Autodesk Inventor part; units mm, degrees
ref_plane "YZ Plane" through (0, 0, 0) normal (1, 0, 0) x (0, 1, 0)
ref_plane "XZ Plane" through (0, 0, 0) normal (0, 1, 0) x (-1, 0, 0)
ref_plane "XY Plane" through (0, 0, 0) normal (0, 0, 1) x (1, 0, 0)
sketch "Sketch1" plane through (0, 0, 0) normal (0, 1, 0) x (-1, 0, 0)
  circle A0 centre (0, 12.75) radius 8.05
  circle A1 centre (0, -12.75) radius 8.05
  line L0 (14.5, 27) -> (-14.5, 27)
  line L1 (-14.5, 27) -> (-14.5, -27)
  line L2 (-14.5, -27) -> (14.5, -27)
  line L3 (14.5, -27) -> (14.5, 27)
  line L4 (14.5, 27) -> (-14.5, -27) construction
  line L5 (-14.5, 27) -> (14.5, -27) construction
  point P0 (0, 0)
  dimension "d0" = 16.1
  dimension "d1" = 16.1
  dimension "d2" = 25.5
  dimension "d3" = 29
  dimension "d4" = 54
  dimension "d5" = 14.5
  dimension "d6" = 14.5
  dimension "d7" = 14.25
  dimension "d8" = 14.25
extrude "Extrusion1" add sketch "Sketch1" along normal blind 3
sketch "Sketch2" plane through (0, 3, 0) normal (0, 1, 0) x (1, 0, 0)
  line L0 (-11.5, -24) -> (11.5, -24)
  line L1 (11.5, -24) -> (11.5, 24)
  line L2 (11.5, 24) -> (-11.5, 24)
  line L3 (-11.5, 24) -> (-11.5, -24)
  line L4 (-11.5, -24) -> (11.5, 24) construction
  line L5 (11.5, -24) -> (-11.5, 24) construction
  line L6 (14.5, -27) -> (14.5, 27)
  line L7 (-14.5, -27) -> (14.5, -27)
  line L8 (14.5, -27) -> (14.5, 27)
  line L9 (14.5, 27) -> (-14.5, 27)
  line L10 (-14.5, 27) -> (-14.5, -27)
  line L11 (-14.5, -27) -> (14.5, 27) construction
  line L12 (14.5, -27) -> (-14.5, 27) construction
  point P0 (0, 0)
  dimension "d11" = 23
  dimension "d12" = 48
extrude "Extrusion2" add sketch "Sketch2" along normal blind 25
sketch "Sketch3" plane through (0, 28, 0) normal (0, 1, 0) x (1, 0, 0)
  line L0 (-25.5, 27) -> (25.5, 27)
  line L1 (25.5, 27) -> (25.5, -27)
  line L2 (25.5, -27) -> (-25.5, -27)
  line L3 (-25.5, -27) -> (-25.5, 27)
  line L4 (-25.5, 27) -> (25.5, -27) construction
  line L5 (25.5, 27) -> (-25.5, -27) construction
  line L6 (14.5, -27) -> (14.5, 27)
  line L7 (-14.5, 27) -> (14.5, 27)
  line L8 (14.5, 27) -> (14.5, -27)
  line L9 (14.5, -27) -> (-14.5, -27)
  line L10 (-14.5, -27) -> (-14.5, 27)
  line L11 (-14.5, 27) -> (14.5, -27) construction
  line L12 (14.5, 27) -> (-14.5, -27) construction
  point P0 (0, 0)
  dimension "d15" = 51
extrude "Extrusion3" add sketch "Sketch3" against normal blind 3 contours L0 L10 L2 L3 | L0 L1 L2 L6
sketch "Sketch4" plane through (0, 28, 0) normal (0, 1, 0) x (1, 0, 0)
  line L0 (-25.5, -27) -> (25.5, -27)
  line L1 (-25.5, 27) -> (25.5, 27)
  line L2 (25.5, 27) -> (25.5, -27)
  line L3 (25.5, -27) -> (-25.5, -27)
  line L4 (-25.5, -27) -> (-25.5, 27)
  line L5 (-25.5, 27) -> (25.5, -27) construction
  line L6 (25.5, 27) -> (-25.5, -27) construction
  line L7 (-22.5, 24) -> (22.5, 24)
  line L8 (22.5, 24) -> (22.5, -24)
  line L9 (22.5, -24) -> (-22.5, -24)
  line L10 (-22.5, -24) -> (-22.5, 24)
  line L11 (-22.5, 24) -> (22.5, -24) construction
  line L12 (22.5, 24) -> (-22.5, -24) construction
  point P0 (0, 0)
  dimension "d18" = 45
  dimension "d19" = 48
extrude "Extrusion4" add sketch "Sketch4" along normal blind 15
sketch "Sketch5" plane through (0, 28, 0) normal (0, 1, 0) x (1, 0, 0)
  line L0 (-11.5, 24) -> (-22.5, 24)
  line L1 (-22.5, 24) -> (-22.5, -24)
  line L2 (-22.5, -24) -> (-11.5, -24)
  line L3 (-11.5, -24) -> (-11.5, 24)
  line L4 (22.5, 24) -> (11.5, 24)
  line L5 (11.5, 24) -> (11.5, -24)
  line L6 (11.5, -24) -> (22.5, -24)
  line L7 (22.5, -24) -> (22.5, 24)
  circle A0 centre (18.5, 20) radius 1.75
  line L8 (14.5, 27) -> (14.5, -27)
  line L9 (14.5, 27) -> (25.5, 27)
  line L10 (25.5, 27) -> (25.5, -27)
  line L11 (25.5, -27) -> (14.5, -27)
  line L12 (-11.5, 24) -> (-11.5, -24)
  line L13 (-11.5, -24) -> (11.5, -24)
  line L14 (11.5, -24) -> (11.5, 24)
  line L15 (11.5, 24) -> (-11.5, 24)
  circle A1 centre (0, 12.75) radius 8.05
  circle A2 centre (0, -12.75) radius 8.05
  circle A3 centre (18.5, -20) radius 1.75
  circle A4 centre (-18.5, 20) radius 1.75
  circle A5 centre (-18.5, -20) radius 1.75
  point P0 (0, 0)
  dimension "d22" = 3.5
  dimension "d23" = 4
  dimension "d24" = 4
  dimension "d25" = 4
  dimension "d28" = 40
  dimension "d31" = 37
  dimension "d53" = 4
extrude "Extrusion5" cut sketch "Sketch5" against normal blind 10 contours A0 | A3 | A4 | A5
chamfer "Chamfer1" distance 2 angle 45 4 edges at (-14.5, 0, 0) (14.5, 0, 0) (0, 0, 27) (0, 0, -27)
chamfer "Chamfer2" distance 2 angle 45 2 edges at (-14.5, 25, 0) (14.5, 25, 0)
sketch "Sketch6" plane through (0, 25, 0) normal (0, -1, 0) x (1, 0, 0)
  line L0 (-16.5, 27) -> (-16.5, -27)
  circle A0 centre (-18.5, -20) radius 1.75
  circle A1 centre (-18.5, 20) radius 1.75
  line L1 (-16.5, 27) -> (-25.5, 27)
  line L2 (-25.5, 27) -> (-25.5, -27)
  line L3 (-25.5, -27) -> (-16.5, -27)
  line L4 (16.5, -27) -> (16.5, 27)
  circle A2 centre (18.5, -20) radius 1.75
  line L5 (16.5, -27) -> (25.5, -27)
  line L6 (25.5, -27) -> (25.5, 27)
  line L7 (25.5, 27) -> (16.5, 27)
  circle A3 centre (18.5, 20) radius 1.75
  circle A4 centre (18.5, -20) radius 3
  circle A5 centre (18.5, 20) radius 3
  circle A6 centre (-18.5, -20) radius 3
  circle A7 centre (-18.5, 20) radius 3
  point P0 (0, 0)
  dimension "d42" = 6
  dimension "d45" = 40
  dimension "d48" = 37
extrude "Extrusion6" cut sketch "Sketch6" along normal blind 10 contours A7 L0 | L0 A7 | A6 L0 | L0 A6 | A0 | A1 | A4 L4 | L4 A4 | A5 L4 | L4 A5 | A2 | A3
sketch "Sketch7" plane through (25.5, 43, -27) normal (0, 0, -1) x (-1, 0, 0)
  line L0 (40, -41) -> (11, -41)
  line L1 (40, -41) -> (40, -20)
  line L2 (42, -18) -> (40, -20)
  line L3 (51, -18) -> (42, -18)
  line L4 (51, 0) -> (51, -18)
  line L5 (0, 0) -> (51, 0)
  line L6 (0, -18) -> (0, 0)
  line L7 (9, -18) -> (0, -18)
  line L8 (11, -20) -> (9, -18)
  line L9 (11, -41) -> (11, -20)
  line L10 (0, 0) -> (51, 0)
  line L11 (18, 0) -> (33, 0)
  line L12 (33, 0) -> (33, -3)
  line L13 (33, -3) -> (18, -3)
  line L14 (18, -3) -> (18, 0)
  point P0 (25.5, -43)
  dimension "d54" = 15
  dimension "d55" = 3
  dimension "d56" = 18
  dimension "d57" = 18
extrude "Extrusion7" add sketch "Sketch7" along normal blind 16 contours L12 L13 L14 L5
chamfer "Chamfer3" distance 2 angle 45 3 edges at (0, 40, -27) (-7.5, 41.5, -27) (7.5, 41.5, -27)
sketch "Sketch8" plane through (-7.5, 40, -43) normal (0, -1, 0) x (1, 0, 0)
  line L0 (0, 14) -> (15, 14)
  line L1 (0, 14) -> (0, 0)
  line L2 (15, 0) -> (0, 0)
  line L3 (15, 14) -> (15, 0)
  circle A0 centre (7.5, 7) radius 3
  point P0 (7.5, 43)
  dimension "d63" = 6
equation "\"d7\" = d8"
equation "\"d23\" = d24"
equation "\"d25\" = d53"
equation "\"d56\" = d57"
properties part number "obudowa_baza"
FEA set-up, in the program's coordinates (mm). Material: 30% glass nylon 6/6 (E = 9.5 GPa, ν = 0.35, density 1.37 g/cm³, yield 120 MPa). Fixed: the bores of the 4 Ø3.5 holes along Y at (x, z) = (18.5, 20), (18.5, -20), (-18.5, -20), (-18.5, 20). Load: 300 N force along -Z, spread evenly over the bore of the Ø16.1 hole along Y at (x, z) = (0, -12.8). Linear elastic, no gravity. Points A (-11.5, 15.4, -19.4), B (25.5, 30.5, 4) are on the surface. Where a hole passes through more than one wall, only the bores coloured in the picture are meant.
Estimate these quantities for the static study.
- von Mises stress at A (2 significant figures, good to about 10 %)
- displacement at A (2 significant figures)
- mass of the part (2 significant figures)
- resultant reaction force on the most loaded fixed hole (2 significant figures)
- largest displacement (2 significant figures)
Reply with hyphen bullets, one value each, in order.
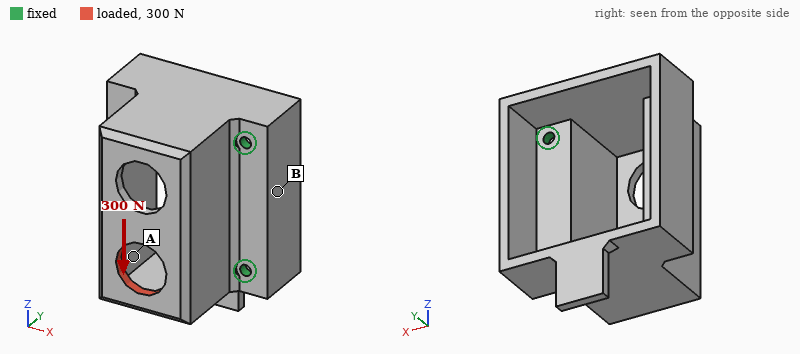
- 1.9 MPa
- 9.3 µm
- 38 g
- 120 N
- 28 µm
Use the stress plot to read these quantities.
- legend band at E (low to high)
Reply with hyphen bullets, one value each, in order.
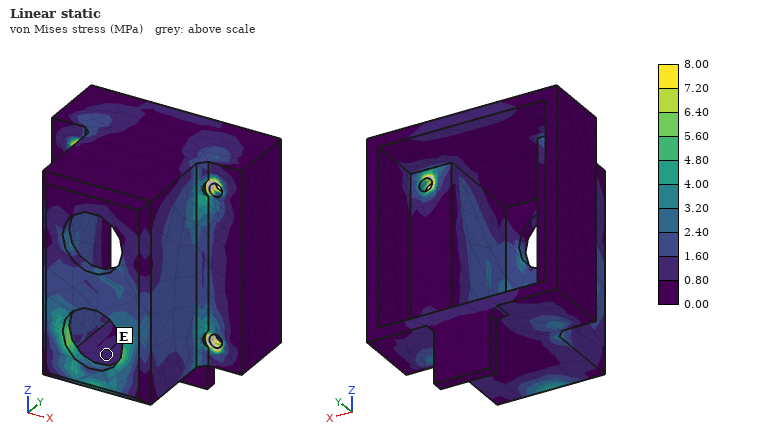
- 0.80 to 1.60 MPa
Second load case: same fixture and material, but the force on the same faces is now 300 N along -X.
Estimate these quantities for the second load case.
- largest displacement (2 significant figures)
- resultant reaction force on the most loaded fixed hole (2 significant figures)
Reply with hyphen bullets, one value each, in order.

- 54 µm
- 170 N
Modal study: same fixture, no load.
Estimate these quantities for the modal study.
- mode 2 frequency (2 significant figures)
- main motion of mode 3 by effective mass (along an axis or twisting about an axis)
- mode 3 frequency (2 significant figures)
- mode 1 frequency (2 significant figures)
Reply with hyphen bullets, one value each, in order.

- 4400 Hz
- along X
- 4700 Hz
- 2700 Hz
